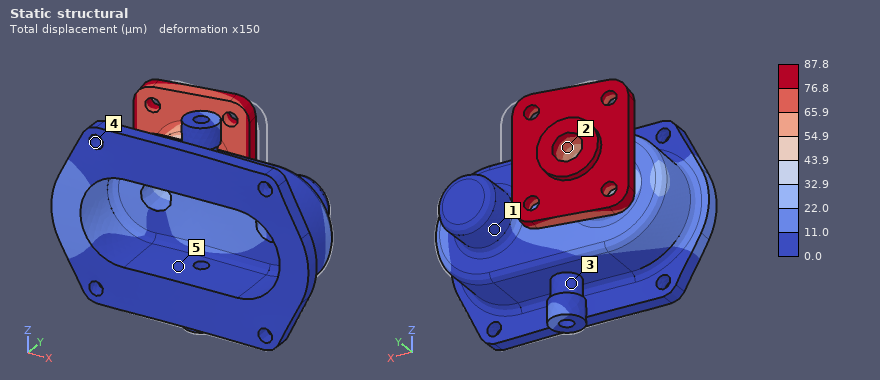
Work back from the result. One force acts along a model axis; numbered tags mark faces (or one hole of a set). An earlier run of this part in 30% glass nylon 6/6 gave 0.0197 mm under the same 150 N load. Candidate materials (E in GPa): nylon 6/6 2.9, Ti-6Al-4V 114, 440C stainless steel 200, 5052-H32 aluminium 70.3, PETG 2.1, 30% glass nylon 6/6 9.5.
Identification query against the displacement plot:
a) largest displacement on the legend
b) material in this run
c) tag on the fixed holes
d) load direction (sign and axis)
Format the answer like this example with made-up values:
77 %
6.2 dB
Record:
87.8 µm
PETG
4
-X
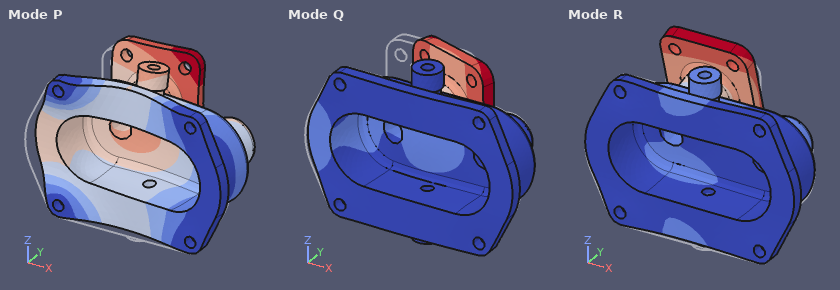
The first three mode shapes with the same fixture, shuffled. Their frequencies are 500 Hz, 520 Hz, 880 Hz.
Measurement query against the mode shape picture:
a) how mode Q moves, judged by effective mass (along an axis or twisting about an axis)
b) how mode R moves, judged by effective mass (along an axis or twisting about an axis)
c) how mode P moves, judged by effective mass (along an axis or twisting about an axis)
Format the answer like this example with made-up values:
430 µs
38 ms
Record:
along X
along Z
along Y
